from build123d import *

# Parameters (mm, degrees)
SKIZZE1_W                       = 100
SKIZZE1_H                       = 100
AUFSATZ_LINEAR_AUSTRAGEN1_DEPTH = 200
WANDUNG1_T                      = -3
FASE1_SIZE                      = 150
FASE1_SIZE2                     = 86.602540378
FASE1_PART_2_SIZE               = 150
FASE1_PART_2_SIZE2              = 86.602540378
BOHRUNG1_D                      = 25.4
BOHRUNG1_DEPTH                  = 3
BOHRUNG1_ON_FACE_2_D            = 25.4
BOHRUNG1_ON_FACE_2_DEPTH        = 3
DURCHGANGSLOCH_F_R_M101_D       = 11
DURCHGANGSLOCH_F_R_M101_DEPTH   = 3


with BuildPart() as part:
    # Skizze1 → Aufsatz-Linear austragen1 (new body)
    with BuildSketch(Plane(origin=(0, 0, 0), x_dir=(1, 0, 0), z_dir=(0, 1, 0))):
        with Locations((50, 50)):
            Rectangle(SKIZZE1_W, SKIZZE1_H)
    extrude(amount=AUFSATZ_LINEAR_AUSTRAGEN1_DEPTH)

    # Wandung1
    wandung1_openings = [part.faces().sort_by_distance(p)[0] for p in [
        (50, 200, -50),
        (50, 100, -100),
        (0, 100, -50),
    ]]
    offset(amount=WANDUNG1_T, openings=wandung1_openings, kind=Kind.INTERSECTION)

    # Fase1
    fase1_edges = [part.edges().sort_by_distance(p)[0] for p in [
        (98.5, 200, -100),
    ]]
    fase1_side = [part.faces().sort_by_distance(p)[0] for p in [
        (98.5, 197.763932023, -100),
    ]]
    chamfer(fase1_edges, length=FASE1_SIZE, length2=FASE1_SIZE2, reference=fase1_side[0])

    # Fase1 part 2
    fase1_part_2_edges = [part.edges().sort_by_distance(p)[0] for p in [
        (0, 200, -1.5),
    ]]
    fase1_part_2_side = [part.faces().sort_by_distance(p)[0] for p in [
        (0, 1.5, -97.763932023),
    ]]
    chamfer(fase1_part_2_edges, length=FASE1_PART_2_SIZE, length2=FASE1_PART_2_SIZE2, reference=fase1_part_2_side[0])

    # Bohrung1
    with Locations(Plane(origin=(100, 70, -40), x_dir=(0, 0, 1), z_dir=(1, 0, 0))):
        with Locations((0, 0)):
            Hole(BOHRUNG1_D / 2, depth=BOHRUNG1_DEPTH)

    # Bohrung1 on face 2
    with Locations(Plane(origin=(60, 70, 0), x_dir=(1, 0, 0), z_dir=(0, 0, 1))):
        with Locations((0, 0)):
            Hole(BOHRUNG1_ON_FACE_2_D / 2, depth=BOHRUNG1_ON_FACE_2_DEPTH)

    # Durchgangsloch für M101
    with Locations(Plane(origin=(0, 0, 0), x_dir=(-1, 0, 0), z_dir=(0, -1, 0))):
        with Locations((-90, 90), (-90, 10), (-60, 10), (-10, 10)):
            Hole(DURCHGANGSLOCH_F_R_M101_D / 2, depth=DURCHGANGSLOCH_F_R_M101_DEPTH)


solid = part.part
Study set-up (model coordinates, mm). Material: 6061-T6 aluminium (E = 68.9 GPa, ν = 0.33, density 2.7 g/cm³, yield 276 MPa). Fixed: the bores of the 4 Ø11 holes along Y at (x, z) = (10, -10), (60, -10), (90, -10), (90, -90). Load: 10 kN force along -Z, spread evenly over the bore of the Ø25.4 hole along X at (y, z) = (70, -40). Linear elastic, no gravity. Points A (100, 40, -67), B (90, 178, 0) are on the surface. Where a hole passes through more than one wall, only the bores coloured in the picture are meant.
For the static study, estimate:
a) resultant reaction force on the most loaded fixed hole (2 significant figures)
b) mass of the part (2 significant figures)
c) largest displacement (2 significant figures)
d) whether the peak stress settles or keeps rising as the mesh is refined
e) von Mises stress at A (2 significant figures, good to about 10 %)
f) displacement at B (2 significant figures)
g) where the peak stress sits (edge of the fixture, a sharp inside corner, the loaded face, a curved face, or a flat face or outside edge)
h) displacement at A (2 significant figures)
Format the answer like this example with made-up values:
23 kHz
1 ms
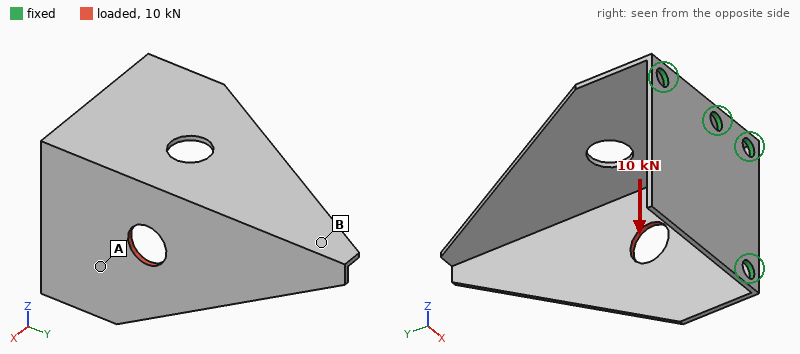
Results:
9.5 kN
280 g
0.61 mm
keeps rising
58 MPa
0.55 mm
edge of the fixture
0.22 mm
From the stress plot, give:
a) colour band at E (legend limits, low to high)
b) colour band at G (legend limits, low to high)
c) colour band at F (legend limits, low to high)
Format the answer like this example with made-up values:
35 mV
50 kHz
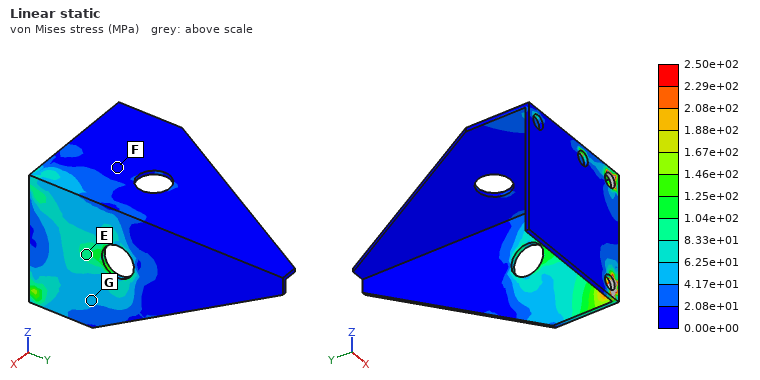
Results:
8.33e+01 to 1.04e+02 MPa
4.17e+01 to 6.25e+01 MPa
0.00e+00 to 2.08e+01 MPa
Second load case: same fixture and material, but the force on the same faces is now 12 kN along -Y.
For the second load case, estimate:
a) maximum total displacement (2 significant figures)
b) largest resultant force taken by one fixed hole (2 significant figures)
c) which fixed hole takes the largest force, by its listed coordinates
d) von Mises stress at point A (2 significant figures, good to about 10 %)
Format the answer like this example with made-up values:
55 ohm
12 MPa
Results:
0.34 mm
7.1 kN
(90, -10)
32 MPa
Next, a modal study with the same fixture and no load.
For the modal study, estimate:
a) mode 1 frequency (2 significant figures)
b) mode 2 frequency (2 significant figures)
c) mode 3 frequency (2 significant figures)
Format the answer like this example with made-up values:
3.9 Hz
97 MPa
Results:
350 Hz
660 Hz
740 Hz
